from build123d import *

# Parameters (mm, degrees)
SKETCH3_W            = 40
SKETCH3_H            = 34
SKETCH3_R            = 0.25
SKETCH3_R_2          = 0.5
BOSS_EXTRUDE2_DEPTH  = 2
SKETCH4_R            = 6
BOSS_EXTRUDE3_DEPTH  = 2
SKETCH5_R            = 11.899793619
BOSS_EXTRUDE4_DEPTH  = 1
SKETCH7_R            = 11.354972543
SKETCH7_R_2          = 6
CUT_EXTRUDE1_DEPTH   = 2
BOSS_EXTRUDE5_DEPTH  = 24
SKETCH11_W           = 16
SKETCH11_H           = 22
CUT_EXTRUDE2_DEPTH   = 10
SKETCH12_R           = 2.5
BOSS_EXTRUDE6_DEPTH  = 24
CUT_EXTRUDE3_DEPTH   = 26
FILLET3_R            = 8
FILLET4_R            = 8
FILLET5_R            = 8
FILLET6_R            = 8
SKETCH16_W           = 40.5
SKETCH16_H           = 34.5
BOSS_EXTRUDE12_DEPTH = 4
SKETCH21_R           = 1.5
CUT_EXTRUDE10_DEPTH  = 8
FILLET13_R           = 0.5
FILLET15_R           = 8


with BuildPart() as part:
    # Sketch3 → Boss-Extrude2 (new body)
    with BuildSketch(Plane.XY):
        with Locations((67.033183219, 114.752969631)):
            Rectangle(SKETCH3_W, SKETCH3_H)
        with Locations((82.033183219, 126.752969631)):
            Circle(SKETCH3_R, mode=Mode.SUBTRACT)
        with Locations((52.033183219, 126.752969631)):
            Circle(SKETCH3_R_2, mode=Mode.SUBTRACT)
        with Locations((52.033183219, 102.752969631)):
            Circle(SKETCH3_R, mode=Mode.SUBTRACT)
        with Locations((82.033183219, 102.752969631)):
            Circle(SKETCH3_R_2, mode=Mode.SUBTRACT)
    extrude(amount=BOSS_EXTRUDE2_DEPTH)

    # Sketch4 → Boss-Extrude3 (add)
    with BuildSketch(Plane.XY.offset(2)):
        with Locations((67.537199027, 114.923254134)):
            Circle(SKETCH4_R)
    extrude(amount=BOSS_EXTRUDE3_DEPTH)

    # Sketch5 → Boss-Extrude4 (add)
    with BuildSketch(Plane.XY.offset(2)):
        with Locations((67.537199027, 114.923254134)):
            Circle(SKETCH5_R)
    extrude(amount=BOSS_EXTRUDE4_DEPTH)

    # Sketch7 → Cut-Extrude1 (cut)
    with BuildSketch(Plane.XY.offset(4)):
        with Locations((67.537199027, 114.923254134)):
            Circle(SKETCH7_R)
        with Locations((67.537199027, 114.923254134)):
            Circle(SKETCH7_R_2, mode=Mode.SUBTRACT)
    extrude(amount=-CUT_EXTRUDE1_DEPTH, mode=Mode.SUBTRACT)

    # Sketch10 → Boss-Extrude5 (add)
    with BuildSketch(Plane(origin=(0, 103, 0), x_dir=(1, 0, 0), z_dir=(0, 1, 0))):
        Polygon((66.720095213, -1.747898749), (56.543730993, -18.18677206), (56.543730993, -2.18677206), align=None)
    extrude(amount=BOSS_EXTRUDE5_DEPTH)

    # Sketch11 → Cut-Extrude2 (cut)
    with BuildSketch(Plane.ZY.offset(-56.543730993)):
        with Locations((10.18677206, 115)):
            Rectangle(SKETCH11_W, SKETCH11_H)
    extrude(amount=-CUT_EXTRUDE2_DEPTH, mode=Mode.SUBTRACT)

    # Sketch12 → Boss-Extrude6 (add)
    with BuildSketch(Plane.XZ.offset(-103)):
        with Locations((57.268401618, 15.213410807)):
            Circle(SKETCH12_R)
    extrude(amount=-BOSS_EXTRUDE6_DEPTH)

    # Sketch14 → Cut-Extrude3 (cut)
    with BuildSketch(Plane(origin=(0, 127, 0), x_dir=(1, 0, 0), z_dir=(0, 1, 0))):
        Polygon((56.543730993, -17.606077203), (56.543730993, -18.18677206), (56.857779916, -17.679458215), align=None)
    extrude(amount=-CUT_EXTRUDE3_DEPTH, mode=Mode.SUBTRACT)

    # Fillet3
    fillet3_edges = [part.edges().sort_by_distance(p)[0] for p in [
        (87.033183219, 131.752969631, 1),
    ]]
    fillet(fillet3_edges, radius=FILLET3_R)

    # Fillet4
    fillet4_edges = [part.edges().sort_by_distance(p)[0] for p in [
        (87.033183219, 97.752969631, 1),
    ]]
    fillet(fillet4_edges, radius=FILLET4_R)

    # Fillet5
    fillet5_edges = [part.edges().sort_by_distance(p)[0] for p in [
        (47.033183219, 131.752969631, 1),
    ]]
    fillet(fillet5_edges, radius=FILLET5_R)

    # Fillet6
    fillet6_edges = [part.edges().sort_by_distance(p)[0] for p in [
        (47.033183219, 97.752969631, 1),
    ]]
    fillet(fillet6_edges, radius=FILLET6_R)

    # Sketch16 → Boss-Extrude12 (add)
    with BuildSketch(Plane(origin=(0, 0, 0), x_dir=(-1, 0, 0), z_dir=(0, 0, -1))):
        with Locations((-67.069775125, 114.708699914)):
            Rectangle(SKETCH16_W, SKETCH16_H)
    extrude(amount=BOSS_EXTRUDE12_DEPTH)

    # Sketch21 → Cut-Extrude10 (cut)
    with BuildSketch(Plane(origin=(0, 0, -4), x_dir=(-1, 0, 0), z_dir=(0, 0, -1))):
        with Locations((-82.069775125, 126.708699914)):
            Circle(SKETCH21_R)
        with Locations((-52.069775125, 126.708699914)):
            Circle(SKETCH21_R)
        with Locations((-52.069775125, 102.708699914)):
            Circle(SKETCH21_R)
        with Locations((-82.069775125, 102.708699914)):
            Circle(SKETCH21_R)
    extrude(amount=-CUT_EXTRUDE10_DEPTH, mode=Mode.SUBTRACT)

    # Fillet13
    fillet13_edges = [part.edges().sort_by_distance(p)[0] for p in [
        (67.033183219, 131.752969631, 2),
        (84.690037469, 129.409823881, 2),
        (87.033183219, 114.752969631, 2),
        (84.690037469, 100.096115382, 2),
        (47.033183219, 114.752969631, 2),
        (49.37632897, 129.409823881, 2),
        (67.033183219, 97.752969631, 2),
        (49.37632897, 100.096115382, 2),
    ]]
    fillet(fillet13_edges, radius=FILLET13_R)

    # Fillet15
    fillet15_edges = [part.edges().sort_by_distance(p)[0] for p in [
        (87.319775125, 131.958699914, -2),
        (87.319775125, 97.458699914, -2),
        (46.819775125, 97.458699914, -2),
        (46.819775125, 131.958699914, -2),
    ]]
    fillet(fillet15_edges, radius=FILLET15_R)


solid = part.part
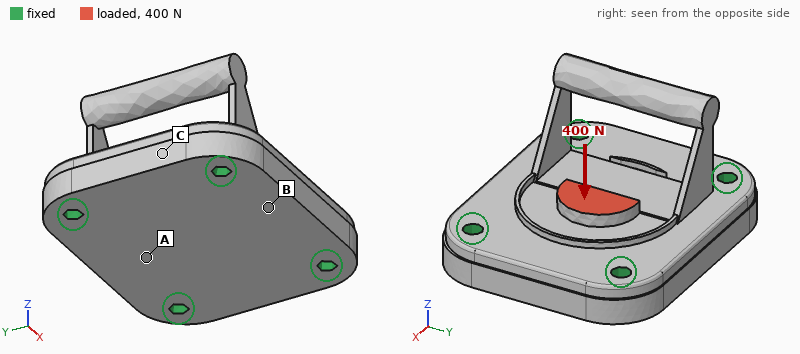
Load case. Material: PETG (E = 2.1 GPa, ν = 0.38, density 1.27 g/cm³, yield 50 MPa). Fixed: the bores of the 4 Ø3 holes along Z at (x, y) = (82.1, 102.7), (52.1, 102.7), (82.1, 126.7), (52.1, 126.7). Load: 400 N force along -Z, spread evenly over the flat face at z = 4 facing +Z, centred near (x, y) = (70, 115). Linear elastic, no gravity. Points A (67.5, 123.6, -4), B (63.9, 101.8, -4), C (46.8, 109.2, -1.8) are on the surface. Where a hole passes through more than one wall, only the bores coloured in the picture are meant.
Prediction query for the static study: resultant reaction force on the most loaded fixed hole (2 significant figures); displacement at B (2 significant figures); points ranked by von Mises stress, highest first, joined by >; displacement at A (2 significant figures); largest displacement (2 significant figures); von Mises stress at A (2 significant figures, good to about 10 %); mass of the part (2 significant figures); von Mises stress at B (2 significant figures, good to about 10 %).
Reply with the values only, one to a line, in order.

120 N
0.043 mm
A > B > C
0.068 mm
0.10 mm
5.4 MPa
11 g
3.1 MPa
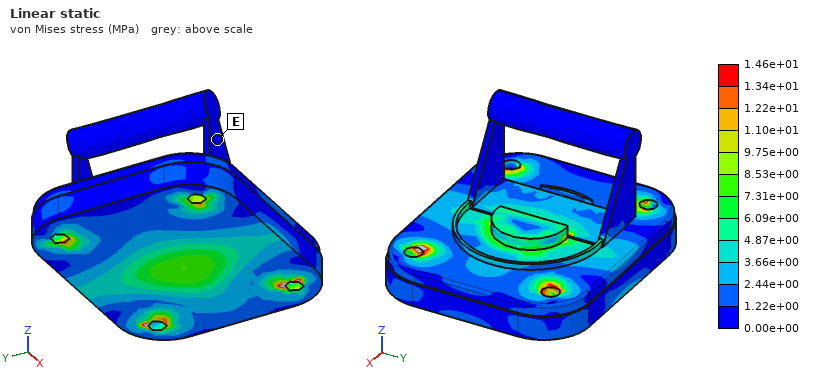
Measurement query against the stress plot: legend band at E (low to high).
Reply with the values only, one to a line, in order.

0.00e+00 to 1.22e+00 MPa
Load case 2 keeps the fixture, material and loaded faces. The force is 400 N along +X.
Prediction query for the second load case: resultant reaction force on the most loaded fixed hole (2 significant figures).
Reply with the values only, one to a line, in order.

120 N
